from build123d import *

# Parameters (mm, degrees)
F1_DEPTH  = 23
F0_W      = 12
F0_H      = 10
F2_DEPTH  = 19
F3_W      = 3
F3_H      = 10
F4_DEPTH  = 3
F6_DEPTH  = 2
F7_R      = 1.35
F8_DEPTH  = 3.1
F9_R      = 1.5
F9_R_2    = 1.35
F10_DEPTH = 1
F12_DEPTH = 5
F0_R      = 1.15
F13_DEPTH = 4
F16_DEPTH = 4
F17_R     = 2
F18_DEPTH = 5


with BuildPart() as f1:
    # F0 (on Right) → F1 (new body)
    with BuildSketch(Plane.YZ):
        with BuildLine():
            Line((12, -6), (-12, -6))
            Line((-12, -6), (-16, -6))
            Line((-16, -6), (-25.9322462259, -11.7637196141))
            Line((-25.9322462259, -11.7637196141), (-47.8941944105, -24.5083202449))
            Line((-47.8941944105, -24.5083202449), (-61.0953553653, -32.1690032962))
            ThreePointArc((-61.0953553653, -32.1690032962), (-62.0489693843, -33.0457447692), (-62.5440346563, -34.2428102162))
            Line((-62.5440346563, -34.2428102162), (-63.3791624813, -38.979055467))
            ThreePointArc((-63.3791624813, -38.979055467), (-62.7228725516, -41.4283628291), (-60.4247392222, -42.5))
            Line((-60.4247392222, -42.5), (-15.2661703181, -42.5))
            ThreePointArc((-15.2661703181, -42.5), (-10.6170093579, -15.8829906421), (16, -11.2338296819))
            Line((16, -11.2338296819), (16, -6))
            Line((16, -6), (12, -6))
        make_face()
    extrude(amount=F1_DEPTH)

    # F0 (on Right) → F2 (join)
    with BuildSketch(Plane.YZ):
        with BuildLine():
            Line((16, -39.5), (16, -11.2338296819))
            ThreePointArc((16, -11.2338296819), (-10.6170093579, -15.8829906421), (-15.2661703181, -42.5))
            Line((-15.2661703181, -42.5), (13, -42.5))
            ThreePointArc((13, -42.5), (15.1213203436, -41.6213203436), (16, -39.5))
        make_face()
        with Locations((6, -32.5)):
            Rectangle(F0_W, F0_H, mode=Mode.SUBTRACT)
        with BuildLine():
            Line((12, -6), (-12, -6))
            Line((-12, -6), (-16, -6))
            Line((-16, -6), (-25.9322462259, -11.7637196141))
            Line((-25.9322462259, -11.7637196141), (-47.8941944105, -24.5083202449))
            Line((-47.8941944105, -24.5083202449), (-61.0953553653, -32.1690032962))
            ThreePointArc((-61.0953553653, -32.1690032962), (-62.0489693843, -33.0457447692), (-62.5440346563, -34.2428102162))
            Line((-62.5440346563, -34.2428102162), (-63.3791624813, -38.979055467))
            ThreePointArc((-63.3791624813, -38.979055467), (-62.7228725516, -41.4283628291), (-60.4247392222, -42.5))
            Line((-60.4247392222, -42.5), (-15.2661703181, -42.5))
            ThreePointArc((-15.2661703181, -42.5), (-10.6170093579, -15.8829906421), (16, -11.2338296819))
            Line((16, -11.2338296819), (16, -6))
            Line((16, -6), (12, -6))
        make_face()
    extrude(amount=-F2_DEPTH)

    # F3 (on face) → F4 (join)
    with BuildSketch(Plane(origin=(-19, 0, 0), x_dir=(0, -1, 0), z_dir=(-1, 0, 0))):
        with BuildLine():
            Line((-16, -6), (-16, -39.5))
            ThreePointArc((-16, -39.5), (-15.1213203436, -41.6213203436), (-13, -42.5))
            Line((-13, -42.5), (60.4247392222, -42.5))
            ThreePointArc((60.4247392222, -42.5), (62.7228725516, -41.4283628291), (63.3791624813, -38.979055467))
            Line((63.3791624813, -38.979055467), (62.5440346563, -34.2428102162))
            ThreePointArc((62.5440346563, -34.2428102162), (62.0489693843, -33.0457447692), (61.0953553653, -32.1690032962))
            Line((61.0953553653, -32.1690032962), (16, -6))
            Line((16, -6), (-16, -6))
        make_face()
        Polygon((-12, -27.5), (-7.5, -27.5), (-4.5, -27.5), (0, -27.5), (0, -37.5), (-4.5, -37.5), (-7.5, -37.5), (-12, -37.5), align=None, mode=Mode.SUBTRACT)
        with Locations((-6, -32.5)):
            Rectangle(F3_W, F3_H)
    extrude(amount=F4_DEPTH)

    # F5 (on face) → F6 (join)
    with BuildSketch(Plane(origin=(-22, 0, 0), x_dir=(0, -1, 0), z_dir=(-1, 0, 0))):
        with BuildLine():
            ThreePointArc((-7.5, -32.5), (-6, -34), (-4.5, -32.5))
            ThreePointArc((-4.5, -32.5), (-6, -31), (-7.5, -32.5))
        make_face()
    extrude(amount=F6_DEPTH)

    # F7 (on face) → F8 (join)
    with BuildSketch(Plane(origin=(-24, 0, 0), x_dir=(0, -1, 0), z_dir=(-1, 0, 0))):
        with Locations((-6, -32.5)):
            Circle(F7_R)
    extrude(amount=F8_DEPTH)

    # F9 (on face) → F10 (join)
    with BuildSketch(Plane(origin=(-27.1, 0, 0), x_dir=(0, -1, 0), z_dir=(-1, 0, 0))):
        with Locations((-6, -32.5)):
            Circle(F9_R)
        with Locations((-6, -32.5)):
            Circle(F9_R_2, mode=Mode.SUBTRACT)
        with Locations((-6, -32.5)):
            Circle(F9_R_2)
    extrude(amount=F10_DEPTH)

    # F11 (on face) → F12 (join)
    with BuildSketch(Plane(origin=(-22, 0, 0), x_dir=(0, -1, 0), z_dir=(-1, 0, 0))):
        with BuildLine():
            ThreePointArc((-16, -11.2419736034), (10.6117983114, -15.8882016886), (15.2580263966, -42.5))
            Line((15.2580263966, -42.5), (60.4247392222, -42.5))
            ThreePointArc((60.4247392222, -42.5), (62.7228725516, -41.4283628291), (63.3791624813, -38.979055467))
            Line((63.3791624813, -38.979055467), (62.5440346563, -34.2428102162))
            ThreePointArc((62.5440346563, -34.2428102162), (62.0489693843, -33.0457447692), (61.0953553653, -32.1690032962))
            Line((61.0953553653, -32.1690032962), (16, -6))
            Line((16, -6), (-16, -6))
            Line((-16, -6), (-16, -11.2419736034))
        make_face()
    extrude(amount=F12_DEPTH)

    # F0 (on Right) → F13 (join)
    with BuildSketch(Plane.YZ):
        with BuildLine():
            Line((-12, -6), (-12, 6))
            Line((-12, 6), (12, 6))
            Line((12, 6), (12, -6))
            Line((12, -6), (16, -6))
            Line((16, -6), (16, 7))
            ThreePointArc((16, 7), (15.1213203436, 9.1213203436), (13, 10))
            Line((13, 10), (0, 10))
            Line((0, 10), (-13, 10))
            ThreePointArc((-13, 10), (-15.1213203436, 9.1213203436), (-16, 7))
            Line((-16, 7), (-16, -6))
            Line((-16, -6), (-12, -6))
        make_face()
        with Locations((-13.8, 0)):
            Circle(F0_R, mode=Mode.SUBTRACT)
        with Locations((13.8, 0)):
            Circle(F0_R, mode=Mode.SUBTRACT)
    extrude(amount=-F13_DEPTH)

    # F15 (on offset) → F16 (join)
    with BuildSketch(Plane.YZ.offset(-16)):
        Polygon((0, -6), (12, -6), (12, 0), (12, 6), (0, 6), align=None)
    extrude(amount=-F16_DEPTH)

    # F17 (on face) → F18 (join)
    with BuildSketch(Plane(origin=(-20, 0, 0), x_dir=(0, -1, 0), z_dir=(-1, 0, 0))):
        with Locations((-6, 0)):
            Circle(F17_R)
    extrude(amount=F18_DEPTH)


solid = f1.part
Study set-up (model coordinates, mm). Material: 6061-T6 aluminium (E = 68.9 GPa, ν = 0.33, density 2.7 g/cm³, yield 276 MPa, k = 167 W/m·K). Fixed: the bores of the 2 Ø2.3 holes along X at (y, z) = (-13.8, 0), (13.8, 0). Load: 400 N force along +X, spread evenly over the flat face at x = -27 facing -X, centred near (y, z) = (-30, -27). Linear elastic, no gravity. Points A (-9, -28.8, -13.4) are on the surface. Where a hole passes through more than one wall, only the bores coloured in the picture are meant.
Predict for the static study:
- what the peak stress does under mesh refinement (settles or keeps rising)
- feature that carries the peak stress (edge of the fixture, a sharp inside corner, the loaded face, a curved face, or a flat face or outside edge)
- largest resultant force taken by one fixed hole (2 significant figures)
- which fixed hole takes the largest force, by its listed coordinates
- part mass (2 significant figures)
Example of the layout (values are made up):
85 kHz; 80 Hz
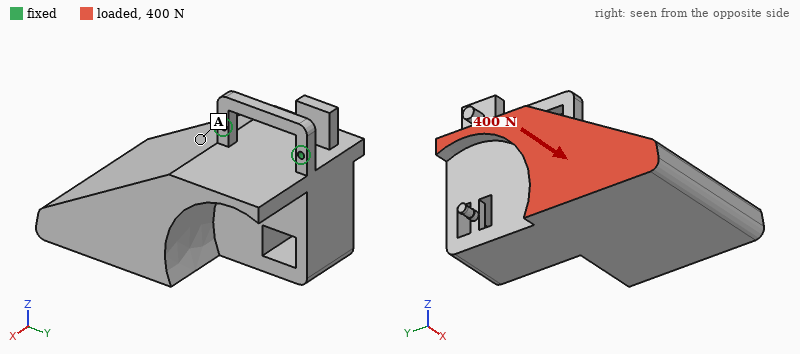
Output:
keeps rising; edge of the fixture; 620 N; (-13.8, 0); 220 g
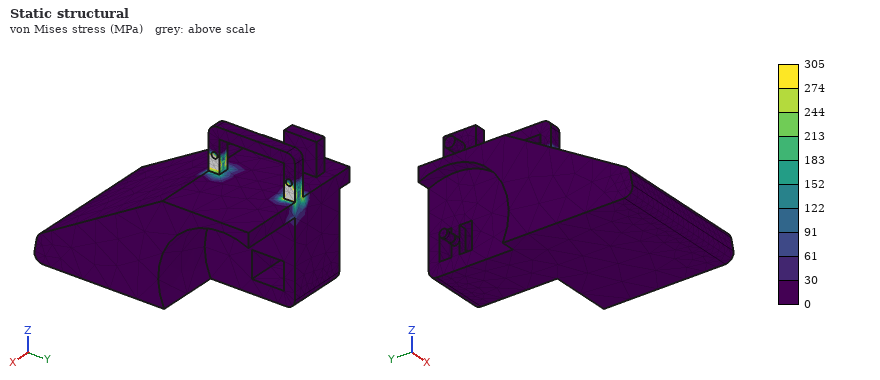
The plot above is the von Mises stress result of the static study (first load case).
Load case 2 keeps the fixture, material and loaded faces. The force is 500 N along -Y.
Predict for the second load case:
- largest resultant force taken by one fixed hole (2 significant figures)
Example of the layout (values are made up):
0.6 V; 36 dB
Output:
650 N
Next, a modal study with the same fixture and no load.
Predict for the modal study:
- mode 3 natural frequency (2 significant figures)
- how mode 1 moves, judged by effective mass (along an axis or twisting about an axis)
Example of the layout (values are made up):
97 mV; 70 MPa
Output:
1600 Hz; along X
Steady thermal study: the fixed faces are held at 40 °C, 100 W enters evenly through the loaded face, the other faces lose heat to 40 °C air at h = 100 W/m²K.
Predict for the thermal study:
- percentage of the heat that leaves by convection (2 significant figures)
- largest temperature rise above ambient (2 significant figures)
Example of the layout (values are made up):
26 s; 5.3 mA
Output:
68 %; 59 K
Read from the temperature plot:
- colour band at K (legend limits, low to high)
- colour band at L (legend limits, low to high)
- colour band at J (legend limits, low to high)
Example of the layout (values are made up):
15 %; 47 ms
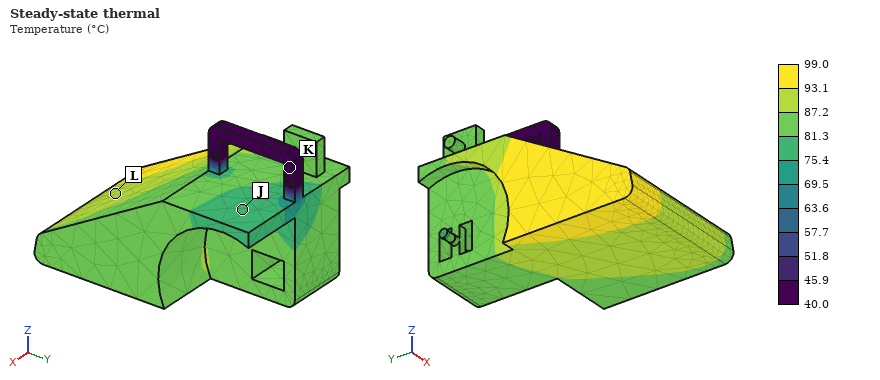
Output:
40.0 to 45.9 °C; 87.2 to 93.1 °C; 75.4 to 81.3 °C
